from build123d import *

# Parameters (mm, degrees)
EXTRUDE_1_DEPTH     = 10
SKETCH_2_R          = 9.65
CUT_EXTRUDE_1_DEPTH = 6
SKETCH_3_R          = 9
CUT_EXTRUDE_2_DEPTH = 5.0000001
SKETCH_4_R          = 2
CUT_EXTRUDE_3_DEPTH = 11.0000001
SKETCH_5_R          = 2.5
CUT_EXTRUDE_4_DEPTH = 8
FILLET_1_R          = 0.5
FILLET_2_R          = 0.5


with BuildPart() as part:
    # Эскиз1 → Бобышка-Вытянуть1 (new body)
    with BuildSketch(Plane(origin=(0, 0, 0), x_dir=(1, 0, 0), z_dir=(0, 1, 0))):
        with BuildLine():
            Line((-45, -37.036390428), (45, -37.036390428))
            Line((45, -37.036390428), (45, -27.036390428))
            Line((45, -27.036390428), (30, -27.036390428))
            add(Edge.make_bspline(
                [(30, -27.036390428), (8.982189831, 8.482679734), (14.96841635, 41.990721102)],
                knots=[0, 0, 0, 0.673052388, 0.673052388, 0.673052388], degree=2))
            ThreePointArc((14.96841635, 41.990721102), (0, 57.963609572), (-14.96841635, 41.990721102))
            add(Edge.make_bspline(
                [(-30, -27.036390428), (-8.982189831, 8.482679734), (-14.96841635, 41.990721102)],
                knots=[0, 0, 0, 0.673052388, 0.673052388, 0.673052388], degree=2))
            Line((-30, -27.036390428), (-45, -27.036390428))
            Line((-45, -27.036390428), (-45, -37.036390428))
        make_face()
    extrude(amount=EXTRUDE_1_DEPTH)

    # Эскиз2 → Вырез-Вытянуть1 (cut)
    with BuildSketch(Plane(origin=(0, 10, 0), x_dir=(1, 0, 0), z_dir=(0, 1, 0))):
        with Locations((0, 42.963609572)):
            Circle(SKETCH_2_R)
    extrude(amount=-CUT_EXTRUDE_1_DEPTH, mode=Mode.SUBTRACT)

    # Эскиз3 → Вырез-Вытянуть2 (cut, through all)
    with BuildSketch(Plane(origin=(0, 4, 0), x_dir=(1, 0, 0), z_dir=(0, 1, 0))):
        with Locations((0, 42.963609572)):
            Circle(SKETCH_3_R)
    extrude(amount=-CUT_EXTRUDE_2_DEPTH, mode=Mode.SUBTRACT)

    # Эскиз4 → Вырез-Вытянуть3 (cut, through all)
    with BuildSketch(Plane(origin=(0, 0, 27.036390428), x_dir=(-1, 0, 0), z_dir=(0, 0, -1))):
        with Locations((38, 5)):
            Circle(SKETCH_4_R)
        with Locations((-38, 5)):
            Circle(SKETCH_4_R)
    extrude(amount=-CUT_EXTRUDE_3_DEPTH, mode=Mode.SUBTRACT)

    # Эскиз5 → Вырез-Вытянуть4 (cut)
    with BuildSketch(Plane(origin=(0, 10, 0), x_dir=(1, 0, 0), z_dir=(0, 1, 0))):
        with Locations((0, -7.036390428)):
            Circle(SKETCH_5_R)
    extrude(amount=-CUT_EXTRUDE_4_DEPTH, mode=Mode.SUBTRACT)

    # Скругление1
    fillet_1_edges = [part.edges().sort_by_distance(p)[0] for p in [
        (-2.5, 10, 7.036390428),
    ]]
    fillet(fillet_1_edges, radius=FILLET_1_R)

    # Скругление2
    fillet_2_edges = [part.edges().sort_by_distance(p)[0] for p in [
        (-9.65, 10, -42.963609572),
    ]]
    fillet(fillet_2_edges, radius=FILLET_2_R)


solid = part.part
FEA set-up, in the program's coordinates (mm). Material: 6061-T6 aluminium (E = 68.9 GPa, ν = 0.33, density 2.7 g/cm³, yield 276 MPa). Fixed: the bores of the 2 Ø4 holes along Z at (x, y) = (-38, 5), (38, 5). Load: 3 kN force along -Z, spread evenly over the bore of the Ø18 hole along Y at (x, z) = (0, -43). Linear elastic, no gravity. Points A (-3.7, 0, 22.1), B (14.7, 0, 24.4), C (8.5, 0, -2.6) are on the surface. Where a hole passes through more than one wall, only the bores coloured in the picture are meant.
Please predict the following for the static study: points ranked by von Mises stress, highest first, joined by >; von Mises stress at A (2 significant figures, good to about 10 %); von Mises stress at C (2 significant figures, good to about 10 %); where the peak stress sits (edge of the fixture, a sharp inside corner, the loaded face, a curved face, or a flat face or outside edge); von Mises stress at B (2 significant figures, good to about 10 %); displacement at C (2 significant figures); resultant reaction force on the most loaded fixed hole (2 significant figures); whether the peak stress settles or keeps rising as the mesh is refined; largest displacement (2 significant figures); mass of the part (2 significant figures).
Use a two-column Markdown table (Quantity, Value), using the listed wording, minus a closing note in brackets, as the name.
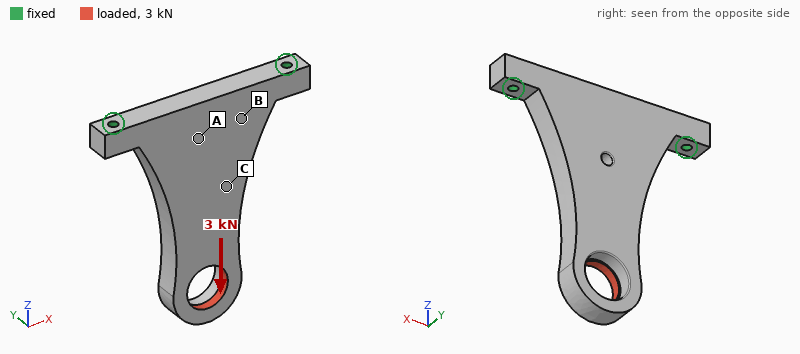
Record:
| Quantity | Value |
|---|---|
| points ranked by von Mises stress, highest first, joined by > | C > B > A |
| von Mises stress at A | 7.7 MPa |
| von Mises stress at C | 24 MPa |
| where the peak stress sits | edge of the fixture |
| von Mises stress at B | 15 MPa |
| displacement at C | 0.081 mm |
| resultant reaction force on the most loaded fixed hole | 1.8 kN |
| whether the peak stress settles or keeps rising as the mesh is refined | keeps rising |
| largest displacement | 0.33 mm |
| mass of the part | 93 g |
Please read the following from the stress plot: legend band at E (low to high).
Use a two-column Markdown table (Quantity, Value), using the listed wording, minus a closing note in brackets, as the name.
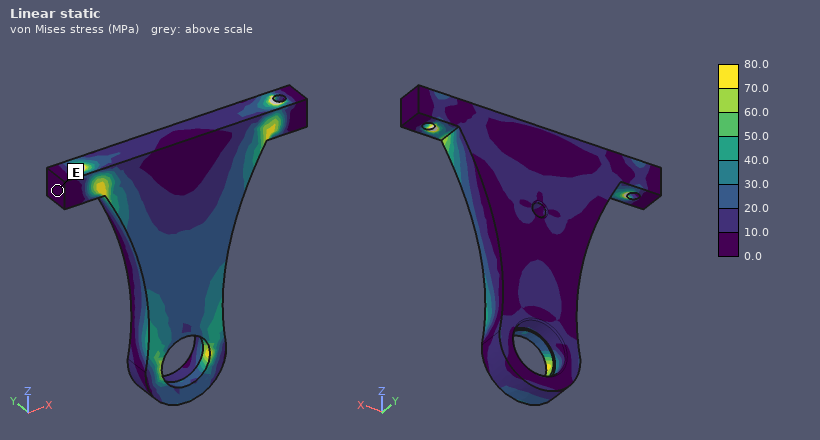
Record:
| Quantity | Value |
|---|---|
| legend band at E | 0.0 to 10.0 MPa |
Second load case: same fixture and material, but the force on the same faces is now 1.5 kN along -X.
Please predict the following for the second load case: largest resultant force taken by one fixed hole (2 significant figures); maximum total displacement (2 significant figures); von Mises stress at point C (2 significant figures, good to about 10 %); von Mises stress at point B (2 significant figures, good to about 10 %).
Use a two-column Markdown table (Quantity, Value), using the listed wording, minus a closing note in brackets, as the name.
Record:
| Quantity | Value |
|---|---|
| largest resultant force taken by one fixed hole | 1.9 kN |
| maximum total displacement | 0.16 mm |
| von Mises stress at point C | 19 MPa |
| von Mises stress at point B | 6.9 MPa |
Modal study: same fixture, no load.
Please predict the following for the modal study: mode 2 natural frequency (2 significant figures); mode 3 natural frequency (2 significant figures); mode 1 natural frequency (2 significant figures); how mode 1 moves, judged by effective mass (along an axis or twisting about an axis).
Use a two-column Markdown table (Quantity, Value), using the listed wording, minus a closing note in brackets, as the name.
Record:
| Quantity | Value |
|---|---|
| mode 2 natural frequency | 4400 Hz |
| mode 3 natural frequency | 4500 Hz |
| mode 1 natural frequency | 860 Hz |
| how mode 1 moves, judged by effective mass | along Y |
